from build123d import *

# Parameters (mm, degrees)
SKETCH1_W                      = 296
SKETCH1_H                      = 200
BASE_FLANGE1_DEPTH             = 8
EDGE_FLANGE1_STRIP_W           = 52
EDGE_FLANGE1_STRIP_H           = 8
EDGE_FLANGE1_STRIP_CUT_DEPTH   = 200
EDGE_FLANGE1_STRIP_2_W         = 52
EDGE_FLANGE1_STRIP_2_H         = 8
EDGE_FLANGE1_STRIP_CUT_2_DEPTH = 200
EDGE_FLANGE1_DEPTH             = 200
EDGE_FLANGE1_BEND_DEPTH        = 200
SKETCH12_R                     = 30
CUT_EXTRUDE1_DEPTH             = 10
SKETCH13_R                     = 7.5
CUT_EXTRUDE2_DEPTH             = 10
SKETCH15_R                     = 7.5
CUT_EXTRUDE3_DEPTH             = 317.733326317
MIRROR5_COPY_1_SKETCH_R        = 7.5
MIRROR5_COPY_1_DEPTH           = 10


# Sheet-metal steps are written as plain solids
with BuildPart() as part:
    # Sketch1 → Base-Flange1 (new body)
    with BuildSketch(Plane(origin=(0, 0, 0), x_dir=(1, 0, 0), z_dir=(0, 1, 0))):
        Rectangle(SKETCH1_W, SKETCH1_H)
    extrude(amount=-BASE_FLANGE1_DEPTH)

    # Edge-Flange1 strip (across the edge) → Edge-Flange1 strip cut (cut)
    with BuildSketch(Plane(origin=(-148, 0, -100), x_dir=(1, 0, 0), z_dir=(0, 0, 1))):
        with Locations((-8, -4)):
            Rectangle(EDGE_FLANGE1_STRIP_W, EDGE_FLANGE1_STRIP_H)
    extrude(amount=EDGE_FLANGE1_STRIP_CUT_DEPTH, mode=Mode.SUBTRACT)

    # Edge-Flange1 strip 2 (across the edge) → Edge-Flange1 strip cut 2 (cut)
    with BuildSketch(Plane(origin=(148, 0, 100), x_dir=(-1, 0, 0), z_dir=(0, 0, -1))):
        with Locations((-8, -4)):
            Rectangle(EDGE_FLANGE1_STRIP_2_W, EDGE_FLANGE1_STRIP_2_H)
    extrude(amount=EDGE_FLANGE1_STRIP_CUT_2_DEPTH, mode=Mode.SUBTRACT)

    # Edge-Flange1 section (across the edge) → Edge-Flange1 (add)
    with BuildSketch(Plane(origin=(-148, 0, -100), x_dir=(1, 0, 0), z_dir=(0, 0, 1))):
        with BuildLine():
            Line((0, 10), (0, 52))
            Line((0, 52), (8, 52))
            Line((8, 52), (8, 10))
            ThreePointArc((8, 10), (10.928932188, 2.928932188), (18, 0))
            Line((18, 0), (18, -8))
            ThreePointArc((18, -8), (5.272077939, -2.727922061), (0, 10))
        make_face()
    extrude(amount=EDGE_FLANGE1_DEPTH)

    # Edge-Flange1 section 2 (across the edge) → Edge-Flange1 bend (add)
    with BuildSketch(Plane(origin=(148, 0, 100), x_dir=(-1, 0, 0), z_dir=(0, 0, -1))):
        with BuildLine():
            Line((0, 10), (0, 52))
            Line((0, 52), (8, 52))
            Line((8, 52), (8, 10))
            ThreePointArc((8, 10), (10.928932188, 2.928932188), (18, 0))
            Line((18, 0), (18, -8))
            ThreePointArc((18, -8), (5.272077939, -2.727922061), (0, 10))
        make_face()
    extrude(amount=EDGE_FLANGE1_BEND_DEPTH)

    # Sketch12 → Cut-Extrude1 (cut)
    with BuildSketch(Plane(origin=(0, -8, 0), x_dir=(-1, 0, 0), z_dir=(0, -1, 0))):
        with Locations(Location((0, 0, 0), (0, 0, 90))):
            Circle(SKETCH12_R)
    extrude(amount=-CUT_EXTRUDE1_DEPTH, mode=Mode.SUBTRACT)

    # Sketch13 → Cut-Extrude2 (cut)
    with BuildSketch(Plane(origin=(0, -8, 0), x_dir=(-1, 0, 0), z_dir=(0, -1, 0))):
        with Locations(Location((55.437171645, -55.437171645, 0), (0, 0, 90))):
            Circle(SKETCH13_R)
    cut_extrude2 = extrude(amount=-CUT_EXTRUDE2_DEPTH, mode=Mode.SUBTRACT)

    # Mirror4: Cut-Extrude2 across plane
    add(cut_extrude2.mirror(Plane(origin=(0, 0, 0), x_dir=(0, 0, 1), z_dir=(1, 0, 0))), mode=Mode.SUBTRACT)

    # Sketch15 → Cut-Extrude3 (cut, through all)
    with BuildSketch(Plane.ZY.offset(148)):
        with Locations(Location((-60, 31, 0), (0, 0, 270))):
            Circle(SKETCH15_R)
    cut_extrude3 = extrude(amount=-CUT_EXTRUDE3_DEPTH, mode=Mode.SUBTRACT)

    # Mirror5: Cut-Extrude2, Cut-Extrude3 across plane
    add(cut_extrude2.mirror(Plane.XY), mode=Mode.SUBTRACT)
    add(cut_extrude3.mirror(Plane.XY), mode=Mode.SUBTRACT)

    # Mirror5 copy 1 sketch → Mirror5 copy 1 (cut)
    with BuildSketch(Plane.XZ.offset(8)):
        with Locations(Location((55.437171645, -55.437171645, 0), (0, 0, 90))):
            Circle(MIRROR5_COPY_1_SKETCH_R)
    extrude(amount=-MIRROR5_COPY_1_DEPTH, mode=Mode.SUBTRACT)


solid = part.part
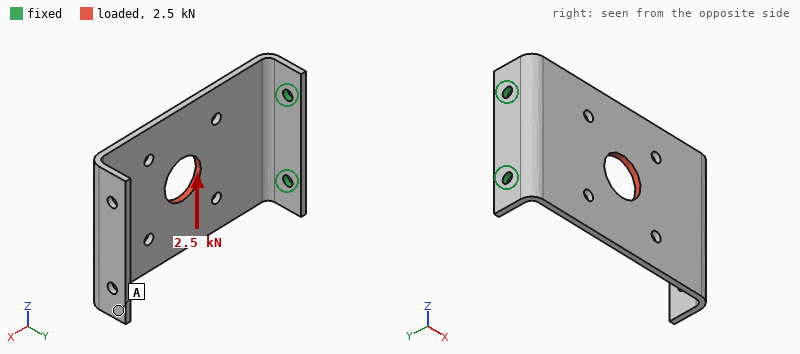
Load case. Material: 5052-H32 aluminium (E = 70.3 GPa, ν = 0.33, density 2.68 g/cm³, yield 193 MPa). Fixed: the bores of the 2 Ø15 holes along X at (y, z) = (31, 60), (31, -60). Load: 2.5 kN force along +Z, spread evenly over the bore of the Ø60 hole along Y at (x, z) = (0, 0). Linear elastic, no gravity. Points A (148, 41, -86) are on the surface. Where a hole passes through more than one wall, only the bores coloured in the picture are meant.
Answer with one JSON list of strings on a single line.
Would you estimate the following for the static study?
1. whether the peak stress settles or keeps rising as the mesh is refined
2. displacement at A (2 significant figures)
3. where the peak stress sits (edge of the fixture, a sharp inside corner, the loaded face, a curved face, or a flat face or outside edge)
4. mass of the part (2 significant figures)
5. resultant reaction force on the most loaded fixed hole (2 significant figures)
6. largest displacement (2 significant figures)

["keeps rising", "0.70 mm", "edge of the fixture", "1.6 kg", "3.1 kN", "0.75 mm"]
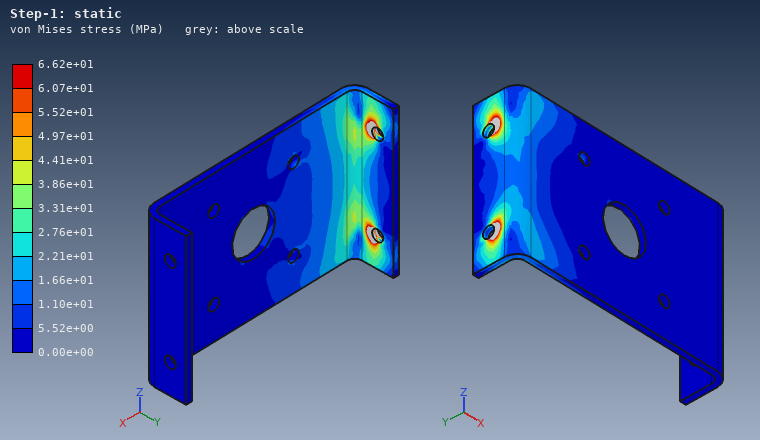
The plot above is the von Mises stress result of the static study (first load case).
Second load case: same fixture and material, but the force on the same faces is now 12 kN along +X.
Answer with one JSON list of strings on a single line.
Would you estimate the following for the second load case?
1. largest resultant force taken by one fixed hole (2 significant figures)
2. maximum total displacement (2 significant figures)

["6.0 kN", "3.8 mm"]
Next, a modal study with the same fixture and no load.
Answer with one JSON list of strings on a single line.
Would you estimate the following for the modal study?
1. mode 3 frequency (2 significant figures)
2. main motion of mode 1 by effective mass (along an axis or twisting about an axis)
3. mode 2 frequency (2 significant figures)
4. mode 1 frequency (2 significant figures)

["330 Hz", "along Y", "180 Hz", "52 Hz"]
